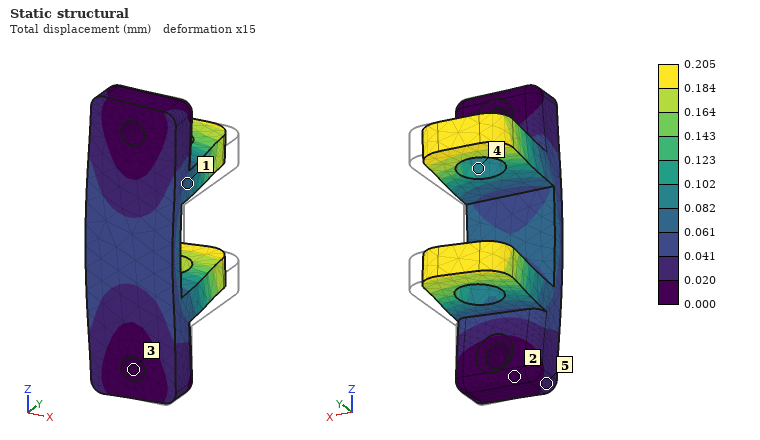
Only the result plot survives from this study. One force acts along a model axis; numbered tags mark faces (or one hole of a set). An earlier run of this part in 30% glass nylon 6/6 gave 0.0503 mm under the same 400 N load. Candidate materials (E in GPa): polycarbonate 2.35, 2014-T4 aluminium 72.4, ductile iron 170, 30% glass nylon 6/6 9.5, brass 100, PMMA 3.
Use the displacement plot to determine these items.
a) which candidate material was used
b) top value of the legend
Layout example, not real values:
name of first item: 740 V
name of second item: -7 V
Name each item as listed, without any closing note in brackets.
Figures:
which candidate material was used: polycarbonate
top value of the legend: 0.205 mm
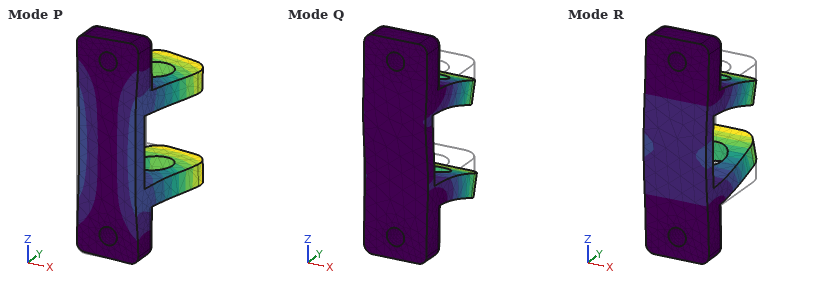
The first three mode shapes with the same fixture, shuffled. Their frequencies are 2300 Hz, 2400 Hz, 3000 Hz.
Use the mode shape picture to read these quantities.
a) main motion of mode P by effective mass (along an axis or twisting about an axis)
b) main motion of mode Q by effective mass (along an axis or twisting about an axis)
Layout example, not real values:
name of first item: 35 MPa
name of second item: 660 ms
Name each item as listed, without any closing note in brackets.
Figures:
main motion of mode P by effective mass: along X
main motion of mode Q by effective mass: along Z
